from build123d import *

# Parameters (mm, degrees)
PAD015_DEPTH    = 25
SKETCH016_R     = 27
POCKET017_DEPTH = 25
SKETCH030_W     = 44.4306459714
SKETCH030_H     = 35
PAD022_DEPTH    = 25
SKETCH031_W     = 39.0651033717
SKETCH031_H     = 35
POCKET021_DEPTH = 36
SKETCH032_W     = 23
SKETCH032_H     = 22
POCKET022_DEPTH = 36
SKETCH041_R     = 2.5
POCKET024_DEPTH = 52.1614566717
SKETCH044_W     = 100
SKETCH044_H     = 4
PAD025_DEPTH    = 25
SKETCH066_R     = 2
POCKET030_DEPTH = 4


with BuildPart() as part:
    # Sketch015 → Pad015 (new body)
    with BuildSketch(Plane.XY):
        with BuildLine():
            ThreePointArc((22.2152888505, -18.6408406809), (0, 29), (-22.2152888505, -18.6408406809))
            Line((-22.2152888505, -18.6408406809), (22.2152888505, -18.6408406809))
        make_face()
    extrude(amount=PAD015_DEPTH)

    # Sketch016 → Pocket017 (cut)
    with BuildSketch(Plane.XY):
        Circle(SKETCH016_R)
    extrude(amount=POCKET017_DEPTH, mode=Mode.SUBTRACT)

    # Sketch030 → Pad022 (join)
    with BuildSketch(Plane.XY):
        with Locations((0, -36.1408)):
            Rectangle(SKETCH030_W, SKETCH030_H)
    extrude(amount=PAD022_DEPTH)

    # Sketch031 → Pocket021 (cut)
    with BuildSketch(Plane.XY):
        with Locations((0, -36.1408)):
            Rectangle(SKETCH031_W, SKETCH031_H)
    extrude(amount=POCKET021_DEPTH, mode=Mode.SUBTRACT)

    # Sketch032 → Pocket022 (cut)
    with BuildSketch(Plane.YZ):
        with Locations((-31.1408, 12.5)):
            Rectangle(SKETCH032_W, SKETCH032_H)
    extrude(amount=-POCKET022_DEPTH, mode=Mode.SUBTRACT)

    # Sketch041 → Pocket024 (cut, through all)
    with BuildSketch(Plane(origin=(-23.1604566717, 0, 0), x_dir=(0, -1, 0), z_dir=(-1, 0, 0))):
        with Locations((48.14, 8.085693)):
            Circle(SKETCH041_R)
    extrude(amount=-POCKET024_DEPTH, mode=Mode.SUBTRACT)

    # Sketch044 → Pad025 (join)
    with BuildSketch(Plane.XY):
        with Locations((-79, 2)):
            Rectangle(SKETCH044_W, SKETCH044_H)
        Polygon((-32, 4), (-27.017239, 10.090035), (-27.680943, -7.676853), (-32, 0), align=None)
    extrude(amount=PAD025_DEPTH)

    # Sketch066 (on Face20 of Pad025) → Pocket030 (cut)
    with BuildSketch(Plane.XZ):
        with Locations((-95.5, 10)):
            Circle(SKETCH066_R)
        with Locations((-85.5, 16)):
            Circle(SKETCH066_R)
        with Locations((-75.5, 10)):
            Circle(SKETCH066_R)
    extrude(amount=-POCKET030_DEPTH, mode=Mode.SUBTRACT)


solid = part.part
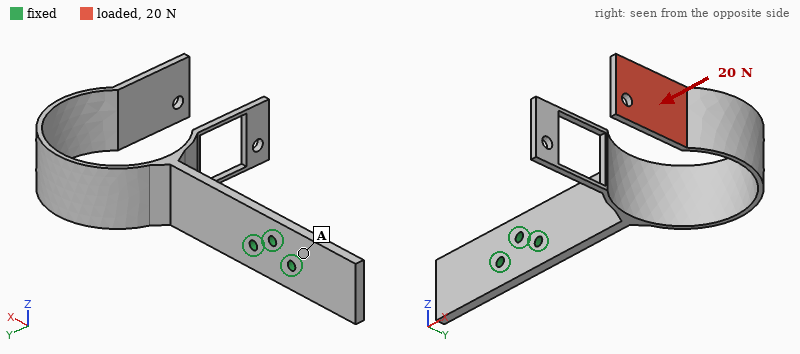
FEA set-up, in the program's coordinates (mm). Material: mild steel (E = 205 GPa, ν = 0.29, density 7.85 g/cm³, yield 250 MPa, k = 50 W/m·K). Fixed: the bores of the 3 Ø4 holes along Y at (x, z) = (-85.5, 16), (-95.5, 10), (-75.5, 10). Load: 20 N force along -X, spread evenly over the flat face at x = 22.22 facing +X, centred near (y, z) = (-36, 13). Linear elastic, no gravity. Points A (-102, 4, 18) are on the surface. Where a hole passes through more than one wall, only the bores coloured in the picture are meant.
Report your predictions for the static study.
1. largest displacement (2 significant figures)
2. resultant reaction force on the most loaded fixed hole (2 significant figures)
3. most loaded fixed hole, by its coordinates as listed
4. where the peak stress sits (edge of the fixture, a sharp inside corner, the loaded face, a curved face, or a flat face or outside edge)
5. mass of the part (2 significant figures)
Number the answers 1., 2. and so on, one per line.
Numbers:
1. 2.1 mm
2. 30 N
3. (-75.5, 10)
4. a curved face
5. 160 g
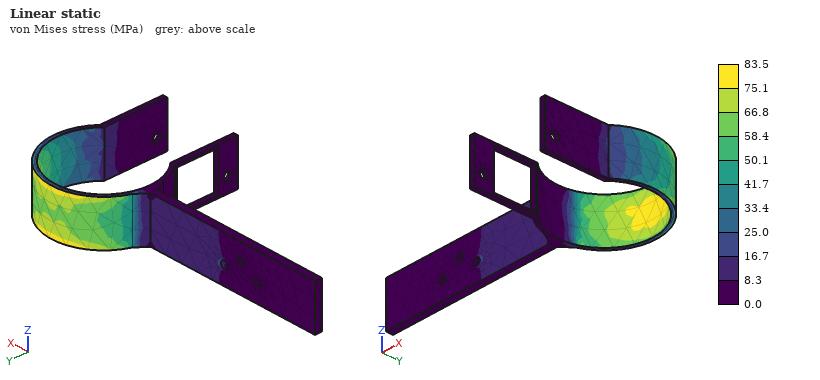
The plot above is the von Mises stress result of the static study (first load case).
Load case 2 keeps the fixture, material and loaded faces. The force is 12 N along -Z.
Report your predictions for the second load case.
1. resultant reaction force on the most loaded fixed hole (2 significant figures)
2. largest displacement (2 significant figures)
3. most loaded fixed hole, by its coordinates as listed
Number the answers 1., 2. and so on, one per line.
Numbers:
1. 65 N
2. 0.67 mm
3. (-75.5, 10)
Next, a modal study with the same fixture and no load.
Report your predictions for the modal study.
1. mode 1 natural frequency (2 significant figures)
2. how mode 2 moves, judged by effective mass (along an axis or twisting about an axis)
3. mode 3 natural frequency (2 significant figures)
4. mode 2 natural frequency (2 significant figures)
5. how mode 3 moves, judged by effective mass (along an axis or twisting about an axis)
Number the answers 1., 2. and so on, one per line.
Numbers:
1. 110 Hz
2. along Z
3. 230 Hz
4. 160 Hz
5. along Y
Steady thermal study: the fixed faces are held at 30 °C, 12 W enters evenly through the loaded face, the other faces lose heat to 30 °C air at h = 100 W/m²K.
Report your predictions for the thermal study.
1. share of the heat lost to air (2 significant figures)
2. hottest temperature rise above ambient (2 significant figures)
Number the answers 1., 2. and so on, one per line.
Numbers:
1. 100 %
2. 66 K
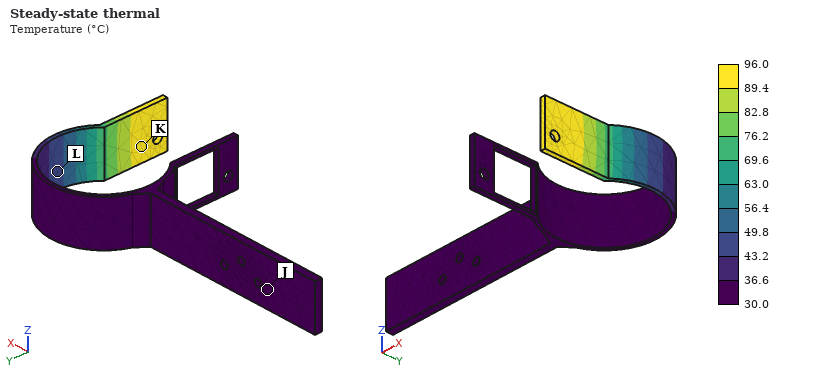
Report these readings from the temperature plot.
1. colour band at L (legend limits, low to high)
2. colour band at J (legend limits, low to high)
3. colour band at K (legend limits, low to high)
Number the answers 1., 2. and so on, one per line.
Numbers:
1. 43.2 to 49.8 °C
2. 30.0 to 36.6 °C
3. 89.4 to 96.0 °C
